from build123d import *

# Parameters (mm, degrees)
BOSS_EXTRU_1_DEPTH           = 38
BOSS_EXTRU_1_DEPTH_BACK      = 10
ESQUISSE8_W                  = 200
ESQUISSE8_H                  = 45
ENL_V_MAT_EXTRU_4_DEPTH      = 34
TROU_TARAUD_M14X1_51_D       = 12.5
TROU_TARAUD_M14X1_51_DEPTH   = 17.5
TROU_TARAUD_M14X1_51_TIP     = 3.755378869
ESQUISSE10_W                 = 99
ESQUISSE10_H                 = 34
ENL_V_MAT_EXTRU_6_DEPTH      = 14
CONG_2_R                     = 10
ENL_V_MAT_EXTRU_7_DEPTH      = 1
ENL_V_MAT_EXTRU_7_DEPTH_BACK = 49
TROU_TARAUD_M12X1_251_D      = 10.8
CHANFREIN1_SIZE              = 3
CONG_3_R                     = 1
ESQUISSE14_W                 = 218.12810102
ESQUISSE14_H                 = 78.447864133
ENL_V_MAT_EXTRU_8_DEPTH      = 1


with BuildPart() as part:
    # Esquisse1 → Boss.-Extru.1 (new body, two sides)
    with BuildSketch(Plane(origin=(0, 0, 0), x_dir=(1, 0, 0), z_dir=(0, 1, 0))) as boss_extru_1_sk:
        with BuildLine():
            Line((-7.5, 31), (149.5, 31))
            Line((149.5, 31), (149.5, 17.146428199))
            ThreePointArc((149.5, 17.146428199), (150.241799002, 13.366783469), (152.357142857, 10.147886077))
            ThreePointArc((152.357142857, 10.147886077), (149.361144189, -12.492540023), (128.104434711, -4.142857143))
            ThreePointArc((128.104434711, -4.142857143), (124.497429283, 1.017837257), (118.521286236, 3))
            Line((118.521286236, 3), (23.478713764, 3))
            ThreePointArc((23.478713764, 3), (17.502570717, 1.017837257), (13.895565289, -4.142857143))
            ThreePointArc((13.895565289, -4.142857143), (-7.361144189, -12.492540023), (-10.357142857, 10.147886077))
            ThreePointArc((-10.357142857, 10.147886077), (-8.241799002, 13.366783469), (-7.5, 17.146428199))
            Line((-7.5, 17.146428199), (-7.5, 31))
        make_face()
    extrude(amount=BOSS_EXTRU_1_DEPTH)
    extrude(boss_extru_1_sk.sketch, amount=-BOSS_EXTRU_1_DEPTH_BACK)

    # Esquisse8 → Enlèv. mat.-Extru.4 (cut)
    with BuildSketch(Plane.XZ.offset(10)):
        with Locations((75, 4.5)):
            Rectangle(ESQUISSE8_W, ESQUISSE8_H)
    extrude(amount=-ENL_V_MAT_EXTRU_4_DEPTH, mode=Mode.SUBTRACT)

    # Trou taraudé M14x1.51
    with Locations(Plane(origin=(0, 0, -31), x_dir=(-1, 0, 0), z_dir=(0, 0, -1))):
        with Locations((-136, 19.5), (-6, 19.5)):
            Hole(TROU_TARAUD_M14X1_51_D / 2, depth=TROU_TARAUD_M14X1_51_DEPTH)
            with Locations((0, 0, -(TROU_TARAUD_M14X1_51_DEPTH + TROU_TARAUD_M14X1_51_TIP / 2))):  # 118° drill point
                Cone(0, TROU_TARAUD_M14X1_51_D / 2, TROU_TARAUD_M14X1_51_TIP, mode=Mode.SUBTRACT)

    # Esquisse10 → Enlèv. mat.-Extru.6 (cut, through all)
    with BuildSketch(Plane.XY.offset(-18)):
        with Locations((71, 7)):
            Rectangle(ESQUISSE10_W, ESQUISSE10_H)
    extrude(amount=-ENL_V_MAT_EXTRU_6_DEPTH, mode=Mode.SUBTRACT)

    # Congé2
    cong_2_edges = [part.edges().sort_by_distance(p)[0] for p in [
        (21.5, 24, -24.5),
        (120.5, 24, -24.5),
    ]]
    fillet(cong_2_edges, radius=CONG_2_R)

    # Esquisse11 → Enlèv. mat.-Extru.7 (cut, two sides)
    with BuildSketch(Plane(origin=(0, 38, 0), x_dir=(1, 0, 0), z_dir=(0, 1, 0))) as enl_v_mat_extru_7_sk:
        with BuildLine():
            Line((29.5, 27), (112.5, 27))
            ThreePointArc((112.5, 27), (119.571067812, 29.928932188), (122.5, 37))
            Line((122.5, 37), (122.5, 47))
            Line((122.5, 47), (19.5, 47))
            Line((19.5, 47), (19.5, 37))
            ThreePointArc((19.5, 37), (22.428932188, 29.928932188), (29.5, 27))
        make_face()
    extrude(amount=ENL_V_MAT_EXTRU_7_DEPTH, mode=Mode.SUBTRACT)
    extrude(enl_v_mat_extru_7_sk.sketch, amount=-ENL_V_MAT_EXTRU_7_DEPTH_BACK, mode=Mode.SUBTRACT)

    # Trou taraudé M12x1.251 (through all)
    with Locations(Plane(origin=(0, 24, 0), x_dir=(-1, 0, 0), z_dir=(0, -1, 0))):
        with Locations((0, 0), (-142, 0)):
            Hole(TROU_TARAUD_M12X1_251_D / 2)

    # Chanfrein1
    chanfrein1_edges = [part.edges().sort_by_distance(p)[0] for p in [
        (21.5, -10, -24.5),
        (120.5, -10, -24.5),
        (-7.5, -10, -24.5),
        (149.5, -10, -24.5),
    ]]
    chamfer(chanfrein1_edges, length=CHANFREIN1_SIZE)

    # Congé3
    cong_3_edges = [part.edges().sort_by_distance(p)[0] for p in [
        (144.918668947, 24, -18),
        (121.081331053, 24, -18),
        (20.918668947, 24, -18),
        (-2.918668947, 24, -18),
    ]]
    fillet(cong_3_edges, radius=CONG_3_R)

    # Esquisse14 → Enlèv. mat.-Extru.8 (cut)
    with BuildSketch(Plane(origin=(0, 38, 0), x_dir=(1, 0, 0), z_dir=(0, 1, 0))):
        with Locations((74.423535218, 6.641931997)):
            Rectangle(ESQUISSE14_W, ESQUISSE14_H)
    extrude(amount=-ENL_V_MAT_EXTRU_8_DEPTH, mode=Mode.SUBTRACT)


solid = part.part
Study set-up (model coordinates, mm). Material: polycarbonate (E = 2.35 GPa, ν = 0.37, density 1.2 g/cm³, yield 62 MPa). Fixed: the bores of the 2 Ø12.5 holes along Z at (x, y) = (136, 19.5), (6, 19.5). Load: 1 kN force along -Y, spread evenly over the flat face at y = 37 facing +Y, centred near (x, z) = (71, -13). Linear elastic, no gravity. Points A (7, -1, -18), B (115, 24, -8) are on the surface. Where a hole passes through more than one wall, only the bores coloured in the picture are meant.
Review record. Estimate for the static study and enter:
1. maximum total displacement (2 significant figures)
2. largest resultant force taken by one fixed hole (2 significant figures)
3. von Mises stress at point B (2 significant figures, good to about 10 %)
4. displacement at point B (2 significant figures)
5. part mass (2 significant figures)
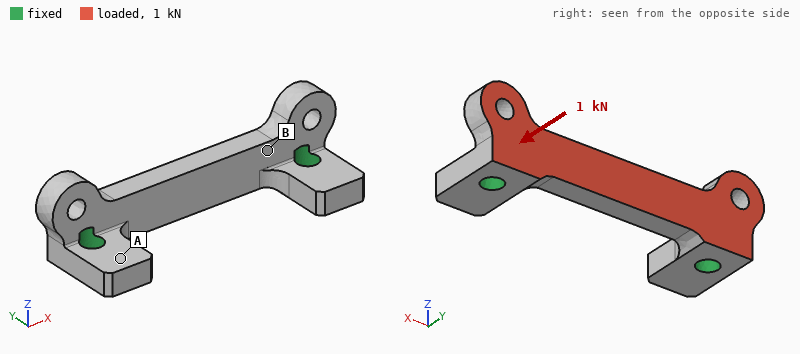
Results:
0.31 mm
520 N
2.1 MPa
0.10 mm
100 g
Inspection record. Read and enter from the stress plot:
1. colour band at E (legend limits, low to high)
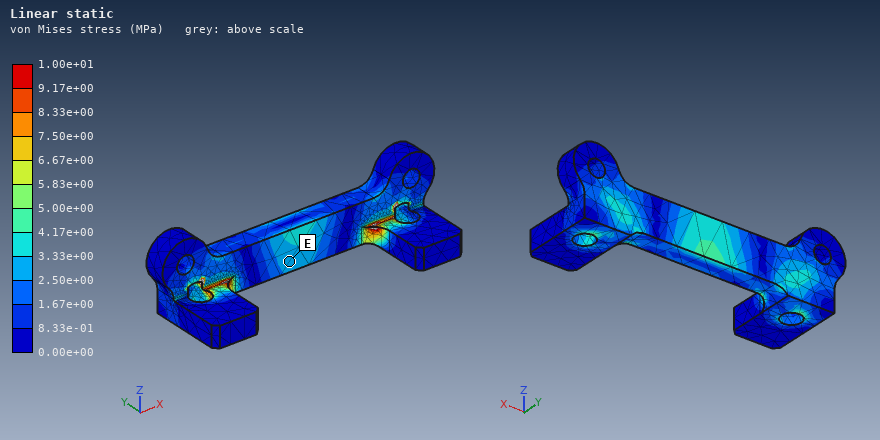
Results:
2.50e+00 to 3.33e+00 MPa
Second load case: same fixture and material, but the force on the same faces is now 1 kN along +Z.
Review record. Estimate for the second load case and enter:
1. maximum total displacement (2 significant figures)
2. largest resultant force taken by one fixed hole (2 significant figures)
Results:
0.24 mm
510 N
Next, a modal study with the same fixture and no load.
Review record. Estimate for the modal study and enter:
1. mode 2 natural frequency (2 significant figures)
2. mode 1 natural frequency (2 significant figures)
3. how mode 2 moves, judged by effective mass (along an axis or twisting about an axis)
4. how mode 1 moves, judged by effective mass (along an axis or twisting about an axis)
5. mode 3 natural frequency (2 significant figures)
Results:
1700 Hz
1300 Hz
along Z
along Y
2200 Hz
